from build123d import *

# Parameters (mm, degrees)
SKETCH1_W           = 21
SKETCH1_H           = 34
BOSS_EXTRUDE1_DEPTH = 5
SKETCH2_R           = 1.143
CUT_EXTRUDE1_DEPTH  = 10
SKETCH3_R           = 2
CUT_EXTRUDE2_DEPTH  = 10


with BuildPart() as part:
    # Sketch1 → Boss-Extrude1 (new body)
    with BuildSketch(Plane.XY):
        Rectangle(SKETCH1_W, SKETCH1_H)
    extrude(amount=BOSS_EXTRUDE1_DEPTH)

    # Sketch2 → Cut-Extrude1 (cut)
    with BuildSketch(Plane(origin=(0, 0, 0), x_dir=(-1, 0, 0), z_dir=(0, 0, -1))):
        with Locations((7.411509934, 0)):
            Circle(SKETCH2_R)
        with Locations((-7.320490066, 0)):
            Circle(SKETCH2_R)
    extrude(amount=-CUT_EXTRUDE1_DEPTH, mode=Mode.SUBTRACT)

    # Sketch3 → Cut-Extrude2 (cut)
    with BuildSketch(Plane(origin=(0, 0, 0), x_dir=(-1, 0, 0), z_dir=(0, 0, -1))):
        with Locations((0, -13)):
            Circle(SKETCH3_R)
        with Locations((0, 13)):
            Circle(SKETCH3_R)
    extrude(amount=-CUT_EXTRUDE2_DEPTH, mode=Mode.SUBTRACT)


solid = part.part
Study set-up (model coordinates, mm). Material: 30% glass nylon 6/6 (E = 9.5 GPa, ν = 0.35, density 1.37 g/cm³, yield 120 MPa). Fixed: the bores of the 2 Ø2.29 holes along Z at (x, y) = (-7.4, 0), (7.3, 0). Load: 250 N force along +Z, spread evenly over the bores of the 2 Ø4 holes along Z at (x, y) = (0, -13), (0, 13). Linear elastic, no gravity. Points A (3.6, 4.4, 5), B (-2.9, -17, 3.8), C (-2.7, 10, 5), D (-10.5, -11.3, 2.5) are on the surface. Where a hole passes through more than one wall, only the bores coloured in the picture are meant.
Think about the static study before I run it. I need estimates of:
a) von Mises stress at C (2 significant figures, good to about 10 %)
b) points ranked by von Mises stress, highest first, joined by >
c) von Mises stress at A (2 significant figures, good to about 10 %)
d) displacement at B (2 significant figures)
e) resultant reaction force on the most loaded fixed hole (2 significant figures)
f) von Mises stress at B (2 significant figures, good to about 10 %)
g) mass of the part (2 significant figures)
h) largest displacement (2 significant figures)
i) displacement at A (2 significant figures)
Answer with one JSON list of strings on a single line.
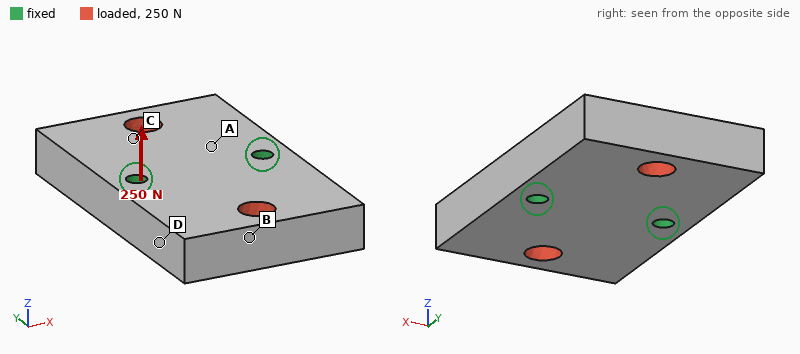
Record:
["7.7 MPa", "A > C > B > D", "12 MPa", "70 µm", "130 N", "4.2 MPa", "4.7 g", "73 µm", "12 µm"]
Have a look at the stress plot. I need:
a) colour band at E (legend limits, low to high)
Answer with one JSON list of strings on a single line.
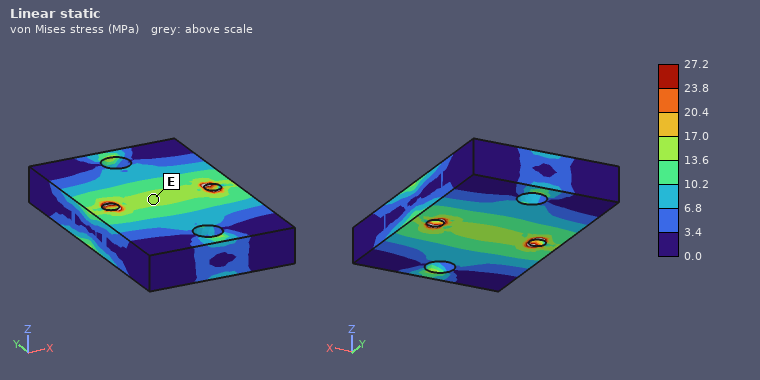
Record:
["13.6 to 17.0 MPa"]
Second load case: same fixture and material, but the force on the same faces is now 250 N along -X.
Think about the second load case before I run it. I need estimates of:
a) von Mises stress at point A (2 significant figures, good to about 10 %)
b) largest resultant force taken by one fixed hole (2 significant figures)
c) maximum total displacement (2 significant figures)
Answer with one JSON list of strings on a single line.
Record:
["2.8 MPa", "130 N", "10 µm"]
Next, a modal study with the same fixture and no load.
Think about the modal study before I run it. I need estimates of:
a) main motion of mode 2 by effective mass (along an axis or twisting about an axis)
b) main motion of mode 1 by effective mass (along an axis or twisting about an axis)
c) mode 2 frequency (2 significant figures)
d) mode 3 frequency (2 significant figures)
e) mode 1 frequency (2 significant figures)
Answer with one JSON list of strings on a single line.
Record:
["along Z", "twisting about X", "7500 Hz", "12 kHz", "6000 Hz"]
